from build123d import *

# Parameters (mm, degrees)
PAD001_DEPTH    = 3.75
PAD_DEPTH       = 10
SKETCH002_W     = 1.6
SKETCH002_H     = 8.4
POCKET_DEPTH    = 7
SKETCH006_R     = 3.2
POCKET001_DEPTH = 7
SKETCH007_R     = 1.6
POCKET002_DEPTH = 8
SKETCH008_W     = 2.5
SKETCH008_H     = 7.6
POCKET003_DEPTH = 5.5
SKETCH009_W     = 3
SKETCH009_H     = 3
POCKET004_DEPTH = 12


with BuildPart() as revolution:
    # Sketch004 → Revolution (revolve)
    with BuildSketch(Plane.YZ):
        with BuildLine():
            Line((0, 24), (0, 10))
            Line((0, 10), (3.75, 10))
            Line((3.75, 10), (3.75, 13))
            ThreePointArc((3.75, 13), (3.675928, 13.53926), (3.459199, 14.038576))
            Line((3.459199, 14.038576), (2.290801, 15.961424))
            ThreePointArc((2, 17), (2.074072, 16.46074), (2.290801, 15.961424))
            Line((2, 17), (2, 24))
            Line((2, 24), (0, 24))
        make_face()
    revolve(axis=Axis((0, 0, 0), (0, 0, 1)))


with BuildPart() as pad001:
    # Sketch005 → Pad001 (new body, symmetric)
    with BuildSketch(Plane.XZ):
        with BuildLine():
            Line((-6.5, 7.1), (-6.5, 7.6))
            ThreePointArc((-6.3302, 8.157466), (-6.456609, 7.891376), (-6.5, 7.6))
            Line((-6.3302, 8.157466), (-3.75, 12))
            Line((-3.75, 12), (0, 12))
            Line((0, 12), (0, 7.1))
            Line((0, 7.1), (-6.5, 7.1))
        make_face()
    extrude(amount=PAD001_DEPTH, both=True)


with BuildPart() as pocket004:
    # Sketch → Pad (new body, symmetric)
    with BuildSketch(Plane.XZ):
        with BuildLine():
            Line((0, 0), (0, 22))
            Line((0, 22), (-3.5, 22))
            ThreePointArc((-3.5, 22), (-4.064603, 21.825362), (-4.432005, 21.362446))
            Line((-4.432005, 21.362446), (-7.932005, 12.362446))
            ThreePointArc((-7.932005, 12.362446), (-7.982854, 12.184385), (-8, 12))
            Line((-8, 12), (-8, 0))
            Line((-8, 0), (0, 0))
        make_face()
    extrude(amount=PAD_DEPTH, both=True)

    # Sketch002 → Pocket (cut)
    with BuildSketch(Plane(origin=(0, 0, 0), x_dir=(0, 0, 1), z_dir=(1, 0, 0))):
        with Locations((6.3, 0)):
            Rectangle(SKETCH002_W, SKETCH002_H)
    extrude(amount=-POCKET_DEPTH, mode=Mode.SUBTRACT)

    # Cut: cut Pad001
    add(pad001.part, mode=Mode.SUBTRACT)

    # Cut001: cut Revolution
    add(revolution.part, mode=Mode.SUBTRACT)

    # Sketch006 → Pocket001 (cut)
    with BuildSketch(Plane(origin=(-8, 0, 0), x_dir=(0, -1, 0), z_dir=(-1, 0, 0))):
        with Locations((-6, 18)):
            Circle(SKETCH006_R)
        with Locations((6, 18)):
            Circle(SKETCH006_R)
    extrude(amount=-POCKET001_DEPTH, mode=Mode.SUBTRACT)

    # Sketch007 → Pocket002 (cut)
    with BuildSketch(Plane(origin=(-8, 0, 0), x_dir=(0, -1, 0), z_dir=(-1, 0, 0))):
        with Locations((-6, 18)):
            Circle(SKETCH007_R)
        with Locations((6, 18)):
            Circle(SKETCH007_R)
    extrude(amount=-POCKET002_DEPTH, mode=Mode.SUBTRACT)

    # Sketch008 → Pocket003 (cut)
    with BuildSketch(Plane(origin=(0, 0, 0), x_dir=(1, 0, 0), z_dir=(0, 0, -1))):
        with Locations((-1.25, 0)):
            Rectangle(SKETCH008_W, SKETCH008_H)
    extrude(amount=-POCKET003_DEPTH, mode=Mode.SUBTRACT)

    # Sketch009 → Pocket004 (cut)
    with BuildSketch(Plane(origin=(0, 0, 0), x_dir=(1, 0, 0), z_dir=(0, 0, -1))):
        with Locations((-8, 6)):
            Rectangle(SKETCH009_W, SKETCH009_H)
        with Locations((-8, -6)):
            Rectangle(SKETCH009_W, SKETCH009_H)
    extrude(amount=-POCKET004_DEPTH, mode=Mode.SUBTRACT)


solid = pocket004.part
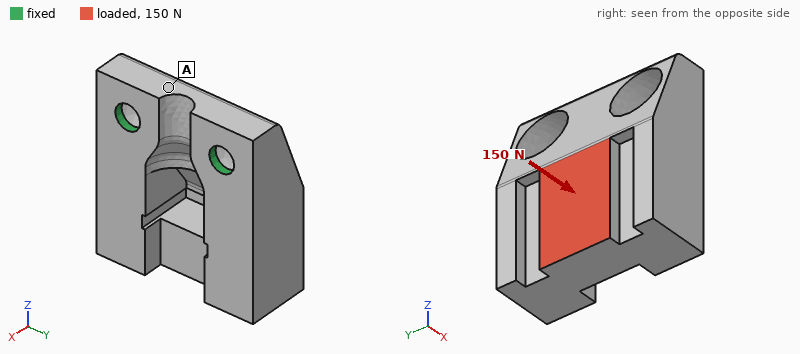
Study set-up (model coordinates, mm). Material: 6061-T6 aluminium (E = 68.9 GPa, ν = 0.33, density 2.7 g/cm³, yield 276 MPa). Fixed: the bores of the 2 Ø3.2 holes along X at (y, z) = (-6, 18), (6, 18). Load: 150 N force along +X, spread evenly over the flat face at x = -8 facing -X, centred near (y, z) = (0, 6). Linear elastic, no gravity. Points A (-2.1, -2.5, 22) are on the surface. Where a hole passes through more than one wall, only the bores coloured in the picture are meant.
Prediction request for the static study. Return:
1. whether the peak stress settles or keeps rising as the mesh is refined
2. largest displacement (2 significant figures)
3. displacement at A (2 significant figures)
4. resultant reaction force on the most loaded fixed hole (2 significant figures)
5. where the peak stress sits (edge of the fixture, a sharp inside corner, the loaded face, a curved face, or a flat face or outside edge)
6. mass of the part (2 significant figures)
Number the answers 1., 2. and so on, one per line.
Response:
1. keeps rising
2. 79 µm
3. 14 µm
4. 77 N
5. edge of the fixture
6. 6.0 g
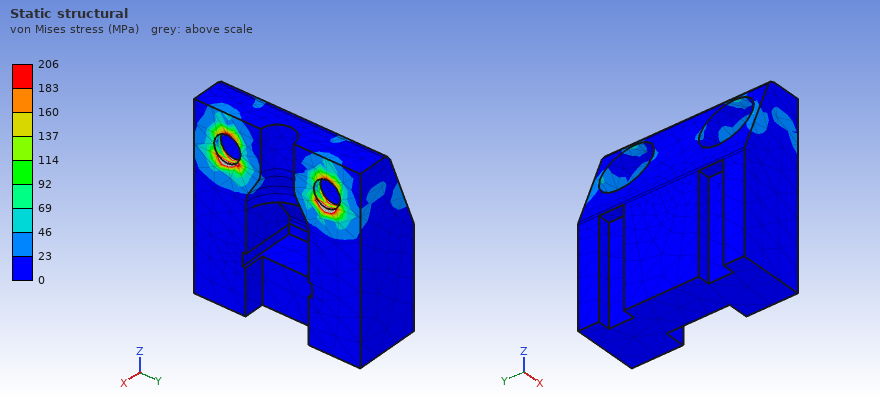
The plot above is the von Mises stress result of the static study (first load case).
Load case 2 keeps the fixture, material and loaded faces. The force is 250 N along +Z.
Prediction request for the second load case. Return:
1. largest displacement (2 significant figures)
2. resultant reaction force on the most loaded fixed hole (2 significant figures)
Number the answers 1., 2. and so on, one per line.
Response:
1. 86 µm
2. 130 N
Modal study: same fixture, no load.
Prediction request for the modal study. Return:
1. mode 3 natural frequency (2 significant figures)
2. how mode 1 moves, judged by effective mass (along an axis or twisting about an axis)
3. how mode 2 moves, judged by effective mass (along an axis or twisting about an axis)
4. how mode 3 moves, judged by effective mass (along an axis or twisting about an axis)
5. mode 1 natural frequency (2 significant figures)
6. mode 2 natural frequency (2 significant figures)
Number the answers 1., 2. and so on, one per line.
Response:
1. 15 kHz
2. along X
3. along Y
4. along Y
5. 3900 Hz
6. 12 kHz
